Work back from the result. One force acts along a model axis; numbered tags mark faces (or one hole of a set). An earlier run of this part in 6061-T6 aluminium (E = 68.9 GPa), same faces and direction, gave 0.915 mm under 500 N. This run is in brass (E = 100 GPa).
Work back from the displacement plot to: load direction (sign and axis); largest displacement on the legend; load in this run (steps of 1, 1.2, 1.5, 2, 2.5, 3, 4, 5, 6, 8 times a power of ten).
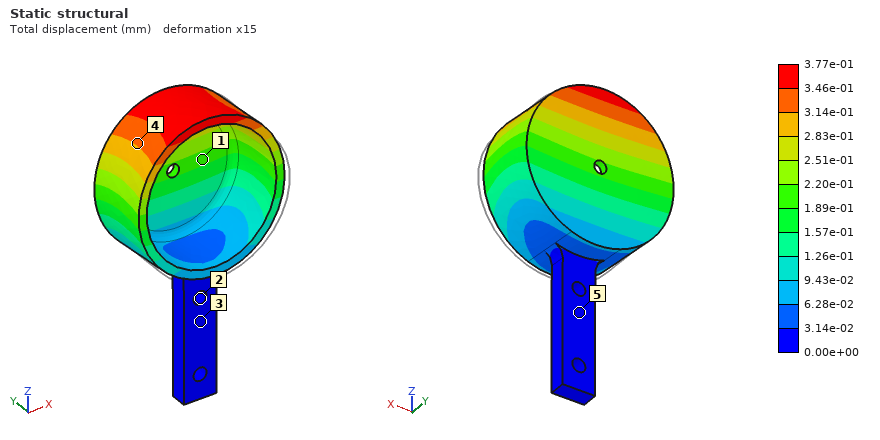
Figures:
+Y
3.77e-01 mm
300 N
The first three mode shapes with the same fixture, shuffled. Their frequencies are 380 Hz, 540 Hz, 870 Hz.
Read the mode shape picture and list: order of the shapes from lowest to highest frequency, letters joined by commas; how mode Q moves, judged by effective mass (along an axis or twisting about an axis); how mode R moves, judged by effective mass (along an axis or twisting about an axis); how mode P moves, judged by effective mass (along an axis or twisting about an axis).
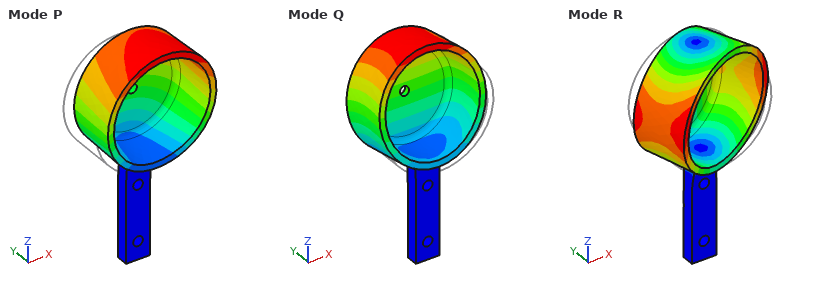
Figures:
Q, P, R
along Y
twisting about Z
along X
